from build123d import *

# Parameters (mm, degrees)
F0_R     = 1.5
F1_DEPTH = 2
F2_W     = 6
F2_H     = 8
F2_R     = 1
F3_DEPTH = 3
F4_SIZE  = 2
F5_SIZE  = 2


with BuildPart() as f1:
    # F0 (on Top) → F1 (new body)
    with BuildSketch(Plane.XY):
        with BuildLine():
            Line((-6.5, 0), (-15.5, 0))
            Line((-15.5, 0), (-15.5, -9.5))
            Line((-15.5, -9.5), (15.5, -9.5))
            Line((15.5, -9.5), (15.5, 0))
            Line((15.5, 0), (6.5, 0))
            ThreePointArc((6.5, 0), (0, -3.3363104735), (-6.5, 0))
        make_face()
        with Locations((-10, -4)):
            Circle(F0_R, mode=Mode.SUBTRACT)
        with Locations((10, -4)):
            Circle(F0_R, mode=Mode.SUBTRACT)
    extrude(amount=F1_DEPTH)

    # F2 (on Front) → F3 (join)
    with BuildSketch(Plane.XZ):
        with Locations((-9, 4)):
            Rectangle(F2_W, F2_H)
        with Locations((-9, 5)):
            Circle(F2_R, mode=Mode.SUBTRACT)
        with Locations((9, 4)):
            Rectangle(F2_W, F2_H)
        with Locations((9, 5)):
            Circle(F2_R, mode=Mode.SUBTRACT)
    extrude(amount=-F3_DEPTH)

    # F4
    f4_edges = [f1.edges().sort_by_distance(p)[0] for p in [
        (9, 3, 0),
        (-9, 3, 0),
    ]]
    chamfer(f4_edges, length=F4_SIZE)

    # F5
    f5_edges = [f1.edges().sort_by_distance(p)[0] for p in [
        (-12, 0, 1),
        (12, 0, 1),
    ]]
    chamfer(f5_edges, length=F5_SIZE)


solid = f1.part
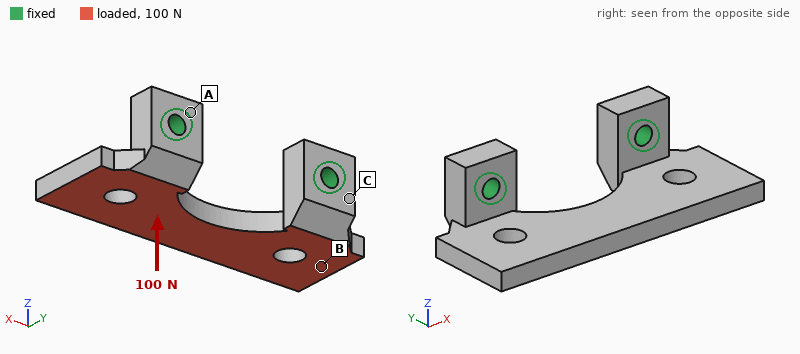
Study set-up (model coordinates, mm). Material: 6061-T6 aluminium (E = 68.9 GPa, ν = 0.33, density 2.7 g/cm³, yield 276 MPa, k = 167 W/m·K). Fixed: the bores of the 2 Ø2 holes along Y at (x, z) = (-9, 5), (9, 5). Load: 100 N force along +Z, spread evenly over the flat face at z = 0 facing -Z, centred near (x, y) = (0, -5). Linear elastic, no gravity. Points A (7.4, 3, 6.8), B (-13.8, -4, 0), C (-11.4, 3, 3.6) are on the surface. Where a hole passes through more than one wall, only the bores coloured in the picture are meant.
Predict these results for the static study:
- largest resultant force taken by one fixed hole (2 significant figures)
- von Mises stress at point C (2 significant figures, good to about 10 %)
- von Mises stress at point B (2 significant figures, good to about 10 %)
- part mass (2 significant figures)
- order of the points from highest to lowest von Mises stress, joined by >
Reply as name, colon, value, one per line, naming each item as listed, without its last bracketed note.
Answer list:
largest resultant force taken by one fixed hole: 50 N
von Mises stress at point C: 25 MPa
von Mises stress at point B: 15 MPa
part mass: 2.0 g
order of the points from highest to lowest von Mises stress, joined by >: C > B > A
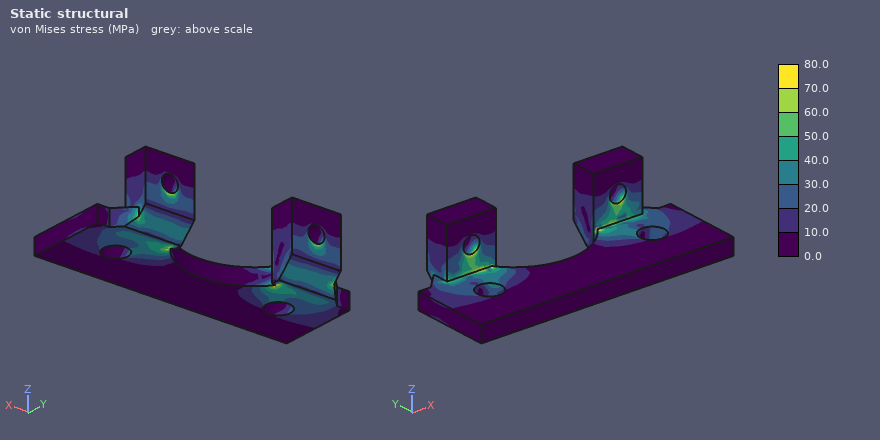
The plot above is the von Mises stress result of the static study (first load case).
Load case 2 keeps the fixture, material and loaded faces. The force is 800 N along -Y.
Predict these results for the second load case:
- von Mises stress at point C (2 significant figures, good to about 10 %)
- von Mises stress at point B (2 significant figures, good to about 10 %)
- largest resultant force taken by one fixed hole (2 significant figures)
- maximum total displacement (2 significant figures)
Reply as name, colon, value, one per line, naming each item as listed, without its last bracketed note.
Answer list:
von Mises stress at point C: 110 MPa
von Mises stress at point B: 41 MPa
largest resultant force taken by one fixed hole: 400 N
maximum total displacement: 0.11 mm
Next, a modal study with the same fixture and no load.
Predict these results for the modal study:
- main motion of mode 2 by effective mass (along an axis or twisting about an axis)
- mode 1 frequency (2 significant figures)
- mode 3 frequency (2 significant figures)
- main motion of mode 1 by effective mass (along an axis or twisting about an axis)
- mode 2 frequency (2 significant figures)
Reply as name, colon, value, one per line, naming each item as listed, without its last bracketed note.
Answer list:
main motion of mode 2 by effective mass: twisting about Y
mode 1 frequency: 7900 Hz
mode 3 frequency: 18 kHz
main motion of mode 1 by effective mass: along Z
mode 2 frequency: 12 kHz
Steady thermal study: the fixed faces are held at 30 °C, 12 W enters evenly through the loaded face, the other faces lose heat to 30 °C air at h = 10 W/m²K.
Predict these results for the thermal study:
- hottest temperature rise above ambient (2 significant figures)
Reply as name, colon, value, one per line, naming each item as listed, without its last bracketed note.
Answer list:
hottest temperature rise above ambient: 21 K
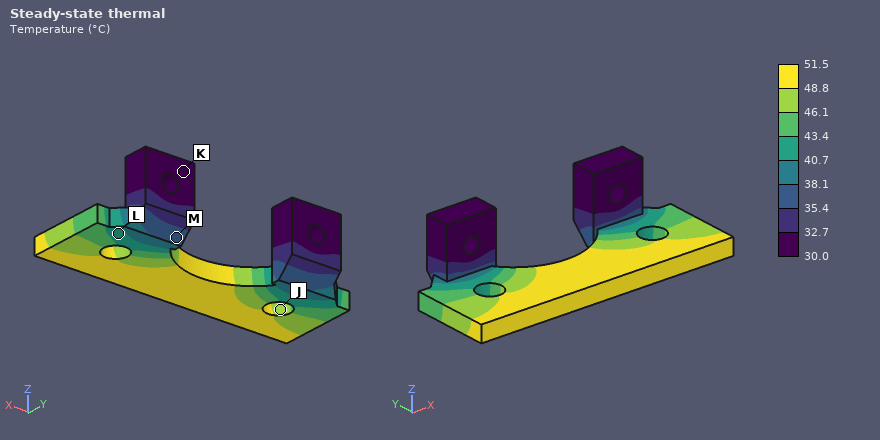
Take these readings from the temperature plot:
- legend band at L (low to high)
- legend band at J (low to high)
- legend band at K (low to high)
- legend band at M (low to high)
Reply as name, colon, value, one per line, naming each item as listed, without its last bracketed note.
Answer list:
legend band at L: 40.7 to 43.4 °C
legend band at J: 46.1 to 48.8 °C
legend band at K: 30.0 to 32.7 °C
legend band at M: 35.4 to 38.1 °C
